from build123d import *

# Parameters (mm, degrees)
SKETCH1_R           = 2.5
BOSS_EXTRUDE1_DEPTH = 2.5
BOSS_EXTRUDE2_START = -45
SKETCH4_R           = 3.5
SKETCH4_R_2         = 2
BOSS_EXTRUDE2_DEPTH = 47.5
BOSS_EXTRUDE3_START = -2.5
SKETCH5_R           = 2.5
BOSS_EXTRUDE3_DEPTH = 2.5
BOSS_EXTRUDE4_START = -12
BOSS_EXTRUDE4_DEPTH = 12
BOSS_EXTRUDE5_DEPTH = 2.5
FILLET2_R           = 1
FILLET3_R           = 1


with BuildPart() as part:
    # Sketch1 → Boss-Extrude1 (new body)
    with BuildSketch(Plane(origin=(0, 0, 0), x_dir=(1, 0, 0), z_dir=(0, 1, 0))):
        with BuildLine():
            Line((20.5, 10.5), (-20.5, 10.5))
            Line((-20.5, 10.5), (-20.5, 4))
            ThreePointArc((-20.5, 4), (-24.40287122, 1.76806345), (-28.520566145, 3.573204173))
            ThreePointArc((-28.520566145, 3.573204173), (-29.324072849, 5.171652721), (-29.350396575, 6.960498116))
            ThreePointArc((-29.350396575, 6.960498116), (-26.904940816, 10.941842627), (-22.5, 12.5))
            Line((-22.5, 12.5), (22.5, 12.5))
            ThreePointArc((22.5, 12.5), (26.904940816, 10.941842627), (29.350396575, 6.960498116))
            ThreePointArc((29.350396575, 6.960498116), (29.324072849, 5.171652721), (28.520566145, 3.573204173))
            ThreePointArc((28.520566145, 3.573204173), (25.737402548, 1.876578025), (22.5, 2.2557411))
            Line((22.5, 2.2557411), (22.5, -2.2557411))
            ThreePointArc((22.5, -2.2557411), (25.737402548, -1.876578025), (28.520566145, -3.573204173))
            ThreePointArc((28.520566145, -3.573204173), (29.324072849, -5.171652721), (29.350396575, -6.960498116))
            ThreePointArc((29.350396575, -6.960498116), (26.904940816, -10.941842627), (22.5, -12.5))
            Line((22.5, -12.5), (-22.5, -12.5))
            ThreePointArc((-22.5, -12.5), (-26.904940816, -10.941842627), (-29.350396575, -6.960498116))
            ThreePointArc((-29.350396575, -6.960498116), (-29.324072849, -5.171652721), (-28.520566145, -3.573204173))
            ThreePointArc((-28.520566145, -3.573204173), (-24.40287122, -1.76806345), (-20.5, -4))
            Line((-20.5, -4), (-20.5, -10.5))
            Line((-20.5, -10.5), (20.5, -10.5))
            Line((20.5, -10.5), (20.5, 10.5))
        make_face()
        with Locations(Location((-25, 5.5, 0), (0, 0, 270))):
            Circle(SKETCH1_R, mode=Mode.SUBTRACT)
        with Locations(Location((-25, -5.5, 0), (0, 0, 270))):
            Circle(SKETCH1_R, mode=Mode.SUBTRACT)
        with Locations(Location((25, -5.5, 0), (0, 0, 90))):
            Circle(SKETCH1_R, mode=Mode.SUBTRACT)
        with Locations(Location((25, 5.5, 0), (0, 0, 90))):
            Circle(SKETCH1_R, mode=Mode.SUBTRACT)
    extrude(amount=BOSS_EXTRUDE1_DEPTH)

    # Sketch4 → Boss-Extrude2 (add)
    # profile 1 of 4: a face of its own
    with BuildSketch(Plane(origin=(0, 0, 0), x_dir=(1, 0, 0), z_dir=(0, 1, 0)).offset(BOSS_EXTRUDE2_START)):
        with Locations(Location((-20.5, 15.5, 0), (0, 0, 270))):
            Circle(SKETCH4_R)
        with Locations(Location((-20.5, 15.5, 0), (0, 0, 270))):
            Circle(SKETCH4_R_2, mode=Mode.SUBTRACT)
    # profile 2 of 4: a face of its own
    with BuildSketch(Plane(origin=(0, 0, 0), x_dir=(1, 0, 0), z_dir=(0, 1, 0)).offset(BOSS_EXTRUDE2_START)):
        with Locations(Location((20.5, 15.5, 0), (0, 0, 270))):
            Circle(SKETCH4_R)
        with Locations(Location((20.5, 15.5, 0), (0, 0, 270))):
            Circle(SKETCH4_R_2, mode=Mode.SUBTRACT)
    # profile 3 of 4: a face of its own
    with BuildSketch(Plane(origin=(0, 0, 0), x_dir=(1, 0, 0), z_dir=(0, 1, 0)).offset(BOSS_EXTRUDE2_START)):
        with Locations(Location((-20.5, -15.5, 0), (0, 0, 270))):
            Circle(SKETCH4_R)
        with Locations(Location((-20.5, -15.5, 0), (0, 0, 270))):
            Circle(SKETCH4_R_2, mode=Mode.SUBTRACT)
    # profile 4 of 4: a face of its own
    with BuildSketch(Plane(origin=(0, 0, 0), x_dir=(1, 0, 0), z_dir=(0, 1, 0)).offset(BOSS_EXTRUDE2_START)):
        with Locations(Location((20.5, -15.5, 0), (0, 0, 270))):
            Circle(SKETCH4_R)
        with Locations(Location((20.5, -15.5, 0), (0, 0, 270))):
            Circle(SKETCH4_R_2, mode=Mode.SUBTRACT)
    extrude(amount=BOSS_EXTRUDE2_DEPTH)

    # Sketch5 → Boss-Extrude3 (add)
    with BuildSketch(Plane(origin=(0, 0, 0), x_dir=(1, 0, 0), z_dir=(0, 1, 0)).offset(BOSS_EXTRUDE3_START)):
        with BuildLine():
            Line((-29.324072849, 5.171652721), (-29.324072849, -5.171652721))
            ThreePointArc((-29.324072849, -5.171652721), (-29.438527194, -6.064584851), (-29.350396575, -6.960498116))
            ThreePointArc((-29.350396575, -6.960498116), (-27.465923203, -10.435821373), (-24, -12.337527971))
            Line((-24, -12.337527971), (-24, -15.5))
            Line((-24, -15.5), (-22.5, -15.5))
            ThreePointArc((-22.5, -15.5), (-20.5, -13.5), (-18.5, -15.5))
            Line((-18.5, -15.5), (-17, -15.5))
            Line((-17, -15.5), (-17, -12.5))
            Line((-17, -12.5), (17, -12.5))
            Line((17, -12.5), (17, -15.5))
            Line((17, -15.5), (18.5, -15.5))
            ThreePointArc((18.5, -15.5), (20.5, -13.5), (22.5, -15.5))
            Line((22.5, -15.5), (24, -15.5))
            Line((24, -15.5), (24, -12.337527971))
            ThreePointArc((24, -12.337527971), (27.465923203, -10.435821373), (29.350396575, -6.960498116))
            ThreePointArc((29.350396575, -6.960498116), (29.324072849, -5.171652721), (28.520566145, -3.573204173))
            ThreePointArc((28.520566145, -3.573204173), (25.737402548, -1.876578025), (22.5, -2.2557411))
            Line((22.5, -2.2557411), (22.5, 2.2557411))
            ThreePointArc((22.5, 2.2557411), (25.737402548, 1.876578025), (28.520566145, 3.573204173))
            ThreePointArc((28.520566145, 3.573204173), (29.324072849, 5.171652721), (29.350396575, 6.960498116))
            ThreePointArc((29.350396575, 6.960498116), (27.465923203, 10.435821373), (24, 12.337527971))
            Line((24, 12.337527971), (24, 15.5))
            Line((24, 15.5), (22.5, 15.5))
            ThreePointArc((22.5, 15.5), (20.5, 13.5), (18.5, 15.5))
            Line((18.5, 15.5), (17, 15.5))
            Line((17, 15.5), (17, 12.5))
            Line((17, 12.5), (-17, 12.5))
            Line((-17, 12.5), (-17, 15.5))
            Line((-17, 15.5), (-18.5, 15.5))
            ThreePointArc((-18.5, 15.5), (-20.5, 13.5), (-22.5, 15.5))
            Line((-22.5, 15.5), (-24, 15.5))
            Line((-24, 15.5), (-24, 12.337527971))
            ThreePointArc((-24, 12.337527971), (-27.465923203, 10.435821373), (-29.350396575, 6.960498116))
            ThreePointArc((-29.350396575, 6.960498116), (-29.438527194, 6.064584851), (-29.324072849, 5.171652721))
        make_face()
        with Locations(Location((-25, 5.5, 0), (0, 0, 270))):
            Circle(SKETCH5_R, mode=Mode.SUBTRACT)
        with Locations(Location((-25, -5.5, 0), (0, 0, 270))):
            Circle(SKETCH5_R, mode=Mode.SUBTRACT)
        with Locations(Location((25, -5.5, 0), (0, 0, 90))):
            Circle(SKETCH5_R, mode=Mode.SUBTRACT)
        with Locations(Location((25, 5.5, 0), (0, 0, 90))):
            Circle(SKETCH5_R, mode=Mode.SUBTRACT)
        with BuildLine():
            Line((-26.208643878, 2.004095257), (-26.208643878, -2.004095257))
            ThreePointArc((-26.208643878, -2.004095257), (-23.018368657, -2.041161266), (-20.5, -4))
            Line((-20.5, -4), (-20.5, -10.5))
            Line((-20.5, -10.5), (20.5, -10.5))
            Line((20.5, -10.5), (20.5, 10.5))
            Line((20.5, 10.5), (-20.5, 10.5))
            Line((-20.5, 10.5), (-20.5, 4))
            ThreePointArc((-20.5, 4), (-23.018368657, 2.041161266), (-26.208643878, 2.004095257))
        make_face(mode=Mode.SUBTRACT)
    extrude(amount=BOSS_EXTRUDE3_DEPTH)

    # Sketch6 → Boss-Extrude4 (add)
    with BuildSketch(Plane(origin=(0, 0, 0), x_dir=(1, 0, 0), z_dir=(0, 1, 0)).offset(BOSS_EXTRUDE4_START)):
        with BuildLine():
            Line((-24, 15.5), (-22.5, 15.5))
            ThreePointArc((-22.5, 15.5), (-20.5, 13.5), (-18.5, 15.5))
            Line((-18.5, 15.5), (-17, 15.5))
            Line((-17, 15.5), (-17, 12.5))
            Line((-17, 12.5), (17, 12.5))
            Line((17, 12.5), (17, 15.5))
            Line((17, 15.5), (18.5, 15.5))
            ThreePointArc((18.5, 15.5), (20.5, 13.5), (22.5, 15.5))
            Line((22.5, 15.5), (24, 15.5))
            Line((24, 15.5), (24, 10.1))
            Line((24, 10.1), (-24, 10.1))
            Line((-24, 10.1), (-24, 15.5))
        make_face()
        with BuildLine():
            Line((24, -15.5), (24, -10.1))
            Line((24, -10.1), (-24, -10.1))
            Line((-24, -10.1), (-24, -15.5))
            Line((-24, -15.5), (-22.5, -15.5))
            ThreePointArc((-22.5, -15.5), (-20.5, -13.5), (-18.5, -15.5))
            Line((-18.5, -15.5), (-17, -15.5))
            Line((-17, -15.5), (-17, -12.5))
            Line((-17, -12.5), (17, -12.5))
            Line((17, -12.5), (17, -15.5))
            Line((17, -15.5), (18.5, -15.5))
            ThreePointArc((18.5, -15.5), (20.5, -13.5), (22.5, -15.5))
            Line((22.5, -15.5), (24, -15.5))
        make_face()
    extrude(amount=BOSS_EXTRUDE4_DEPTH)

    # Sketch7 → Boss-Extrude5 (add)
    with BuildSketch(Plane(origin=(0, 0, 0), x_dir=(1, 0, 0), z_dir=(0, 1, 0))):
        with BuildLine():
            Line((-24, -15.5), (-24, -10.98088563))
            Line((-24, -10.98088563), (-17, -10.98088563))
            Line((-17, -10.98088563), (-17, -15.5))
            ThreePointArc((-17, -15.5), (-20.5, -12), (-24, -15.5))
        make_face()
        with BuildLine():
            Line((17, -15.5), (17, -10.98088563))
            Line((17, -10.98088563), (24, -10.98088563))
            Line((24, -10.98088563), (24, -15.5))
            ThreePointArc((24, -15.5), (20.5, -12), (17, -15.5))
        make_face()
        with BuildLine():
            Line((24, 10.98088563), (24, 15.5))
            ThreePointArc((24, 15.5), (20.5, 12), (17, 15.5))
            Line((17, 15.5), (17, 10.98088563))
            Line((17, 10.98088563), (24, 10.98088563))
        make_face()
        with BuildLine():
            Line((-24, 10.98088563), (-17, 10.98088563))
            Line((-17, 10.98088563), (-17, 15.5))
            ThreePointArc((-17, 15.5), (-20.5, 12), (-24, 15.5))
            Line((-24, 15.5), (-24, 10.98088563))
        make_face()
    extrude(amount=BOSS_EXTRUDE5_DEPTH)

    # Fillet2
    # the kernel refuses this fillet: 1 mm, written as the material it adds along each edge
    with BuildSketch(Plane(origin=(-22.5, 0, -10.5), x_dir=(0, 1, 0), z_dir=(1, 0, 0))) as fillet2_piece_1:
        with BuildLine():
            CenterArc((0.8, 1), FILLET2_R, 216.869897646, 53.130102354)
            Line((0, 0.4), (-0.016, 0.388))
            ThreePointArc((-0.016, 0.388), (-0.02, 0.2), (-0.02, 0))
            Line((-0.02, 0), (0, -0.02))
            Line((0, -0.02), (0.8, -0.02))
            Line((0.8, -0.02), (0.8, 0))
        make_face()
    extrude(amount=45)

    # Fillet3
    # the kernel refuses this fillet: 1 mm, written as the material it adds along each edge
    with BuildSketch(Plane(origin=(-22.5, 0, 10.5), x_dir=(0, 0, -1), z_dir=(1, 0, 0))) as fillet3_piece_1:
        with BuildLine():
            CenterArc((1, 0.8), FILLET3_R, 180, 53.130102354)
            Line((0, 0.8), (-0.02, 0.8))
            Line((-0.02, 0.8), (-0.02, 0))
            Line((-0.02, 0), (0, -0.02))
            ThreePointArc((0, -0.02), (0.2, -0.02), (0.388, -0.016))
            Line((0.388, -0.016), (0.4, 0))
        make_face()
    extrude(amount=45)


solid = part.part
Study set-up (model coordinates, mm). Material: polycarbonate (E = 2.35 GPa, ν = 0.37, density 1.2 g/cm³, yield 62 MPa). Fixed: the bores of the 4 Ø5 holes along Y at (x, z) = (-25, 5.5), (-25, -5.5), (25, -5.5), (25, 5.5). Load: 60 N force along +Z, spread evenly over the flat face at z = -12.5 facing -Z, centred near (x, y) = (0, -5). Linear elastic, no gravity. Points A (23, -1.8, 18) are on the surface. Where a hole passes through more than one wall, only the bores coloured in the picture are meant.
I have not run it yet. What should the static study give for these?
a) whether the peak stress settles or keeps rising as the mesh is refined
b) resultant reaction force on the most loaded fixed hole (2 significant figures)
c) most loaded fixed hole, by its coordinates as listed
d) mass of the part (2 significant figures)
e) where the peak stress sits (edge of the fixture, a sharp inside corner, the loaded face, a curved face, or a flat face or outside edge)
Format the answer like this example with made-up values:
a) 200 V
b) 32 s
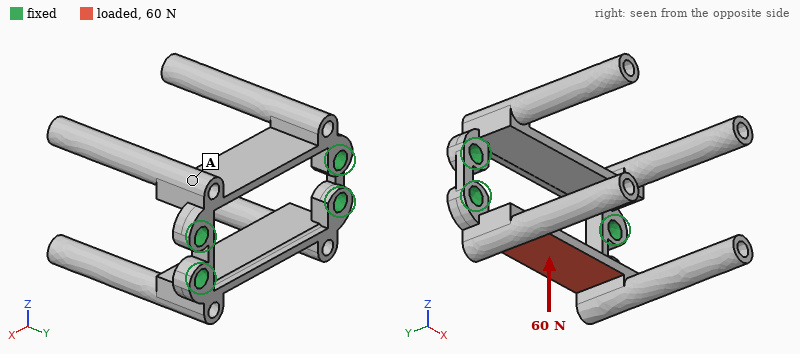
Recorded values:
a) keeps rising
b) 34 N
c) (-25, -5.5)
d) 11 g
e) a sharp inside corner
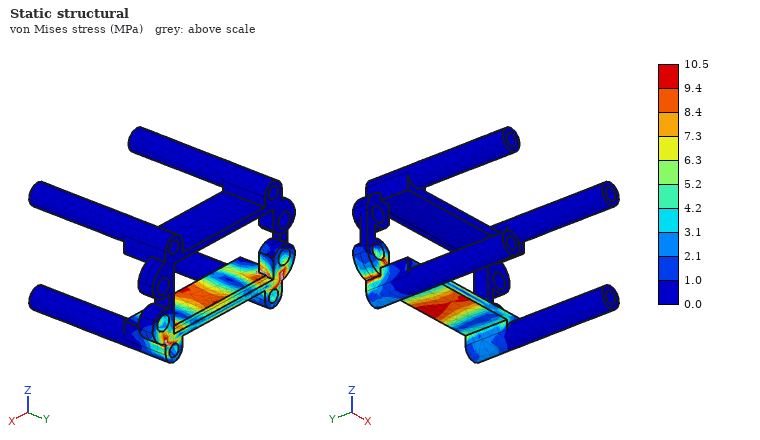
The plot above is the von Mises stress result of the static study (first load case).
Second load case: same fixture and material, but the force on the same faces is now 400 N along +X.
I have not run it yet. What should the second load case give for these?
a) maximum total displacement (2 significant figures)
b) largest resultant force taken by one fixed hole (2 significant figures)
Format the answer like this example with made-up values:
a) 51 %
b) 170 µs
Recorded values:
a) 0.24 mm
b) 210 N
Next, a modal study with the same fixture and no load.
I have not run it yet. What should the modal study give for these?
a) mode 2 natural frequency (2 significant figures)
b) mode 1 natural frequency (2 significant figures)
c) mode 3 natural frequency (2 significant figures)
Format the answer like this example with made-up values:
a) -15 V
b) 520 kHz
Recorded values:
a) 600 Hz
b) 600 Hz
c) 640 Hz
